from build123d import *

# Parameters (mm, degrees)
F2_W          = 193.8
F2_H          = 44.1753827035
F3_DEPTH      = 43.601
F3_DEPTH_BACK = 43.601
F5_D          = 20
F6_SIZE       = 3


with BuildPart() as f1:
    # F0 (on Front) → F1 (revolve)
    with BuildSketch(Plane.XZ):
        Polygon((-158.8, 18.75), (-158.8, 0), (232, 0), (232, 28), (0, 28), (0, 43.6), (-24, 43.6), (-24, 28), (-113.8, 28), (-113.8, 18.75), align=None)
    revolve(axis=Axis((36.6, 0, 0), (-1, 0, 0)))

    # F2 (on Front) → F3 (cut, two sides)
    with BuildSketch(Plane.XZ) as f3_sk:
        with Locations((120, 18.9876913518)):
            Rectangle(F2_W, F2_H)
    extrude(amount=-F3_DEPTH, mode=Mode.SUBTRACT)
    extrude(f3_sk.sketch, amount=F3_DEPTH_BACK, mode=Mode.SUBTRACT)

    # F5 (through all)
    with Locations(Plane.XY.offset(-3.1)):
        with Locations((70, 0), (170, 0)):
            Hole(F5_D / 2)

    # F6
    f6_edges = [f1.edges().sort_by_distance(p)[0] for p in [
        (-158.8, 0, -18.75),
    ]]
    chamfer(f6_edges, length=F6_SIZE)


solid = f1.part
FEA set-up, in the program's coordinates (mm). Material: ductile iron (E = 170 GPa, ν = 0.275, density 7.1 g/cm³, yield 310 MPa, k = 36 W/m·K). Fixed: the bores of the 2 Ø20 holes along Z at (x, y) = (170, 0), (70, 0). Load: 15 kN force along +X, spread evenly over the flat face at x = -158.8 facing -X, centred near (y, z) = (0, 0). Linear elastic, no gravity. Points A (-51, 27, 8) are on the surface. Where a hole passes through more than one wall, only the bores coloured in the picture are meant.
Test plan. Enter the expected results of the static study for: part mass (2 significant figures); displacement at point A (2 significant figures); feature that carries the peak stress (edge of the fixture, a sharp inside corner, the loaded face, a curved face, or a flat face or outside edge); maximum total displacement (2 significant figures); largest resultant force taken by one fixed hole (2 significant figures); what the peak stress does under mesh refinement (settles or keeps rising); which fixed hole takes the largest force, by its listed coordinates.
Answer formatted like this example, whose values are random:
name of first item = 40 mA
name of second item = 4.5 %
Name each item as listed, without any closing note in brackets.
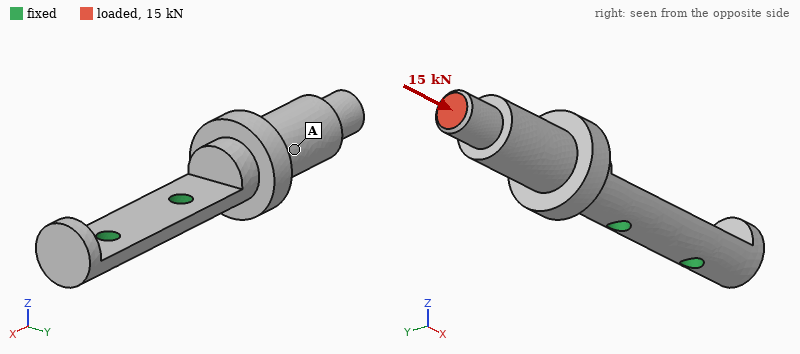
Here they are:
part mass = 5.0 kg
displacement at point A = 0.13 mm
feature that carries the peak stress = edge of the fixture
maximum total displacement = 0.27 mm
largest resultant force taken by one fixed hole = 14 kN
what the peak stress does under mesh refinement = keeps rising
which fixed hole takes the largest force, by its listed coordinates = (70, 0)
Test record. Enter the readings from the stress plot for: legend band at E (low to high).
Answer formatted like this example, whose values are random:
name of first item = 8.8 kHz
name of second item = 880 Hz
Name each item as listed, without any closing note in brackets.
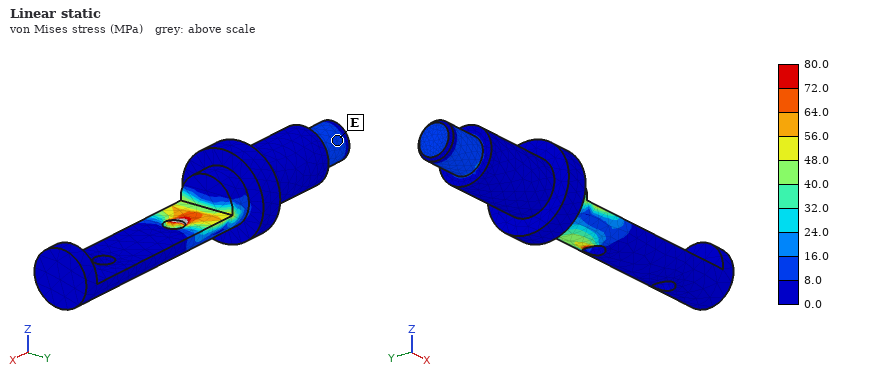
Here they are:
legend band at E = 8.0 to 16.0 MPa
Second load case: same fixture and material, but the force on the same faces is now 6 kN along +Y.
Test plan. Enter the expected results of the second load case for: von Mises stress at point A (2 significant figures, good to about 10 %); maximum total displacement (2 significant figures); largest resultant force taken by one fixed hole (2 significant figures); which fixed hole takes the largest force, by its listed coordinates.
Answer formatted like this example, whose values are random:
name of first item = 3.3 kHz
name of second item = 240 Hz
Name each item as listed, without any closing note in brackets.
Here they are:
von Mises stress at point A = 36 MPa
maximum total displacement = 0.63 mm
largest resultant force taken by one fixed hole = 10.0 kN
which fixed hole takes the largest force, by its listed coordinates = (70, 0)
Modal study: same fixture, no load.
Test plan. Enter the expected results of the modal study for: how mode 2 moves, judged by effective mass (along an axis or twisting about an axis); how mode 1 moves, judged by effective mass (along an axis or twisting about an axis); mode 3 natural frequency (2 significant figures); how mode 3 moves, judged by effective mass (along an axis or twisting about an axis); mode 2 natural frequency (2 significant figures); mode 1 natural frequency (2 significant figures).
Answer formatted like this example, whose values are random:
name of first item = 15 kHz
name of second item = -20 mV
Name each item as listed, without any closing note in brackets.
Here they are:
how mode 2 moves, judged by effective mass = along Y
how mode 1 moves, judged by effective mass = along Z
mode 3 natural frequency = 1500 Hz
how mode 3 moves, judged by effective mass = twisting about X
mode 2 natural frequency = 540 Hz
mode 1 natural frequency = 330 Hz
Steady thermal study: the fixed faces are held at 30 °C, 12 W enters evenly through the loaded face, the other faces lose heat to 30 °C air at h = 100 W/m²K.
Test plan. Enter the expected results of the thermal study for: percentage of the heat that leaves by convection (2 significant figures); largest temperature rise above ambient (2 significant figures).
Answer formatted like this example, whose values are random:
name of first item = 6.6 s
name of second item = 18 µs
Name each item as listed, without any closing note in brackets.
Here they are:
percentage of the heat that leaves by convection = 96 %
largest temperature rise above ambient = 17 K
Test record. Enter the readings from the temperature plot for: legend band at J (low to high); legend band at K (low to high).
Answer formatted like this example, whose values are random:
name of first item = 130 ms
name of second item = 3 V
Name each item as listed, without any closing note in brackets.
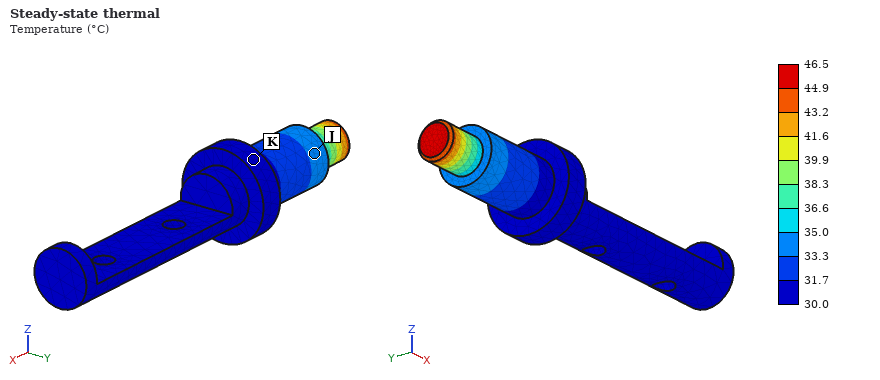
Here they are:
legend band at J = 33.3 to 35.0 °C
legend band at K = 30.0 to 31.7 °C
